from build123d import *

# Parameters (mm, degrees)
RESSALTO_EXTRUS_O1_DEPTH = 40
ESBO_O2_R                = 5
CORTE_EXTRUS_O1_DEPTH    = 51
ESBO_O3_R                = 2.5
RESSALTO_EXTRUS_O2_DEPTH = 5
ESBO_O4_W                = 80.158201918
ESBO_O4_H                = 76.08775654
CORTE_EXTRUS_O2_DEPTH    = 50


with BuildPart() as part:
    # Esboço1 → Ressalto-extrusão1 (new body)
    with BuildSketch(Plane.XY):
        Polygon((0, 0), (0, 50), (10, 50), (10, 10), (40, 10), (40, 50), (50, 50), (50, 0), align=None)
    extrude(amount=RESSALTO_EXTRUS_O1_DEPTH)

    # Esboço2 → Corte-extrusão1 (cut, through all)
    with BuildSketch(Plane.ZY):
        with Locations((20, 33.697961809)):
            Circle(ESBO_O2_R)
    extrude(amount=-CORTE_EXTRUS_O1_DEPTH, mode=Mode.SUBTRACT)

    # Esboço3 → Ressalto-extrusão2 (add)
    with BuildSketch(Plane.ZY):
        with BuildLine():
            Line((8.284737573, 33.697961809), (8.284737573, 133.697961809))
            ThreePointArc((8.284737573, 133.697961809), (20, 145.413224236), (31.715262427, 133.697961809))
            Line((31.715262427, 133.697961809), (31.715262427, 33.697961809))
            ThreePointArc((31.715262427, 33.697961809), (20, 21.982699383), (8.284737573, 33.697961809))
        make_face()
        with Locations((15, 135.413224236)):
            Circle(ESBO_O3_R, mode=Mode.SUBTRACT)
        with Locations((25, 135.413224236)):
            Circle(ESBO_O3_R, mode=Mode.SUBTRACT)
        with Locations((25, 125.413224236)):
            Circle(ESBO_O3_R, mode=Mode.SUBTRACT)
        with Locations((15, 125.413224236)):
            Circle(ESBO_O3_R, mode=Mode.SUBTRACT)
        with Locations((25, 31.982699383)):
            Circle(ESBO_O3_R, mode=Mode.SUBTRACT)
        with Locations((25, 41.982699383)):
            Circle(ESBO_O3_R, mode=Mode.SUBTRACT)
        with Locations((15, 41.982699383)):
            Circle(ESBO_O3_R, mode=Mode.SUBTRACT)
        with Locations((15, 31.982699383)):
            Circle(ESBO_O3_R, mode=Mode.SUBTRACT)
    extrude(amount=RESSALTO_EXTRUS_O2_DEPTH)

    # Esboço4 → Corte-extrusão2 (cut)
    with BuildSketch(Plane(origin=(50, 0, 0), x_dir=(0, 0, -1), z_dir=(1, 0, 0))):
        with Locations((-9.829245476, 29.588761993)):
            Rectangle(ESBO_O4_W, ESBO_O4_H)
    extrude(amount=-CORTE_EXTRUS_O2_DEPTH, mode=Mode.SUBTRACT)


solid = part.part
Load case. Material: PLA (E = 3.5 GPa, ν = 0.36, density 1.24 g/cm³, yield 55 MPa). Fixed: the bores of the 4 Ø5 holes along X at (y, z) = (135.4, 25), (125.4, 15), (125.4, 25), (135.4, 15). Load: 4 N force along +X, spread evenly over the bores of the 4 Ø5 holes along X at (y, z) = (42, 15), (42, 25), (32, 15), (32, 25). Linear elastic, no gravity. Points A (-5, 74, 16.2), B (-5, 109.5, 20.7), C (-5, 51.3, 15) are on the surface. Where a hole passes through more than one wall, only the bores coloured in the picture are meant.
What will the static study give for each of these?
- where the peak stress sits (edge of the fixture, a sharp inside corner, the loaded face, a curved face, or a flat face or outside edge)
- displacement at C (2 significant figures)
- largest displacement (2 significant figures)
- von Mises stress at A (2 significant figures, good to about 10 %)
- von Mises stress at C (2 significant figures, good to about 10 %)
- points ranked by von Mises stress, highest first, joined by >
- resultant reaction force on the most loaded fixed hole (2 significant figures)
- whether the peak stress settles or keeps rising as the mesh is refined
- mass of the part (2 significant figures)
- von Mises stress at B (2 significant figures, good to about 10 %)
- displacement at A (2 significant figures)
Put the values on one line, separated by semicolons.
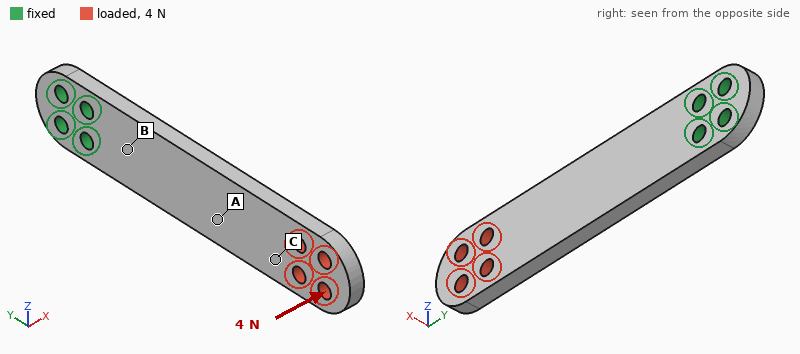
edge of the fixture; 0.76 mm; 1.3 mm; 1.5 MPa; 0.60 MPa; B > A > C; 3.7 N; keeps rising; 16 g; 2.8 MPa; 0.40 mm
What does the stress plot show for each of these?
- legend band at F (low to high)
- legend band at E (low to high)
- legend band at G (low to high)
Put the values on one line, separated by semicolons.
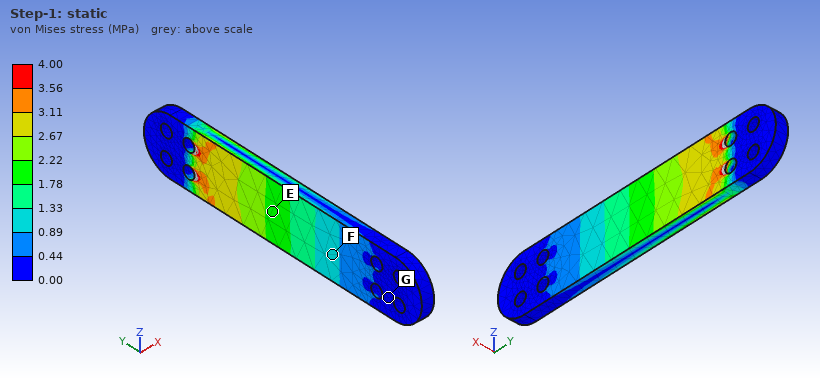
0.89 to 1.33 MPa; 1.78 to 2.22 MPa; 0.00 to 0.44 MPa
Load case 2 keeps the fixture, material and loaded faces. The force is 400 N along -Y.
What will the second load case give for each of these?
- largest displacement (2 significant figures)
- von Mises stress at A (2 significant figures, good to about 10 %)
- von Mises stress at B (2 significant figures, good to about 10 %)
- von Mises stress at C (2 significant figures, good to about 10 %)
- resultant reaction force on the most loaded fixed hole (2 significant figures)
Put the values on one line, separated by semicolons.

93 µm; 3.4 MPa; 3.6 MPa; 3.3 MPa; 190 N
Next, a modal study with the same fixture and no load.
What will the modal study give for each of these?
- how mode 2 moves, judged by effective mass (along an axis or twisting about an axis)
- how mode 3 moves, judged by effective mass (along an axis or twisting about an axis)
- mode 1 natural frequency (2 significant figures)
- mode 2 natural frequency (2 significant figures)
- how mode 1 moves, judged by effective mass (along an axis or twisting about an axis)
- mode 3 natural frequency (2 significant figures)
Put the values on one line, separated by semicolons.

along Z; along X; 150 Hz; 610 Hz; along X; 860 Hz
